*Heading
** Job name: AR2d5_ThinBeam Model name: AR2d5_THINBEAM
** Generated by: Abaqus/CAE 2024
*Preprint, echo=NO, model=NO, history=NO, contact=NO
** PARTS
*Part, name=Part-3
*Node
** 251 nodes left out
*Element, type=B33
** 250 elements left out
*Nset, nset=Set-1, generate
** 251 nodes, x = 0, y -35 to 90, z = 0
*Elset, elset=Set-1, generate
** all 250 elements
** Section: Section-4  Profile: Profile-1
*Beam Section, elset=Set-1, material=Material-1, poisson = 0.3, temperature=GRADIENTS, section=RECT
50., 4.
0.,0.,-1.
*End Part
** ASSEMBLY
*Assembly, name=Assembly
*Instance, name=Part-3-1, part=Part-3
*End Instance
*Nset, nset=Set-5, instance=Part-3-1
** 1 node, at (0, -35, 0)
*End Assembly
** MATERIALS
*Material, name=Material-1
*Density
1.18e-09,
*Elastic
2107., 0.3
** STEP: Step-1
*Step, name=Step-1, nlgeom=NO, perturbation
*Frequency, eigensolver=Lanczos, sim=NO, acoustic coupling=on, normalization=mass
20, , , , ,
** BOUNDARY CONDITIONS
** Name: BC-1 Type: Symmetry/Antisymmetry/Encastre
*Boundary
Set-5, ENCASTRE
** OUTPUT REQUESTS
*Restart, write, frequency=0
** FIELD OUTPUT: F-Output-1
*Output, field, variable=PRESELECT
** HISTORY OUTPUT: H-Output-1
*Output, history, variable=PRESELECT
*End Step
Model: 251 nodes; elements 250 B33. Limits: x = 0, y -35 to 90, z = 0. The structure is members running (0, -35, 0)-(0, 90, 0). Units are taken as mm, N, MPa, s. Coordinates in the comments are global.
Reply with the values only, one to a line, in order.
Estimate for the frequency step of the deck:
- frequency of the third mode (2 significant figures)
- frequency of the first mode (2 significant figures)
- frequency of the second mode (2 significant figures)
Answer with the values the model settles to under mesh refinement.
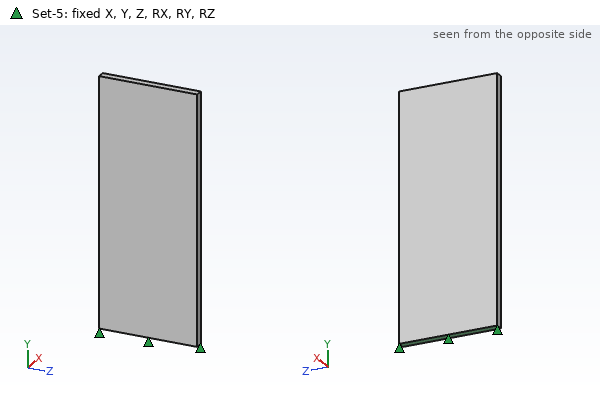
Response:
350 Hz
57 Hz
260 Hz
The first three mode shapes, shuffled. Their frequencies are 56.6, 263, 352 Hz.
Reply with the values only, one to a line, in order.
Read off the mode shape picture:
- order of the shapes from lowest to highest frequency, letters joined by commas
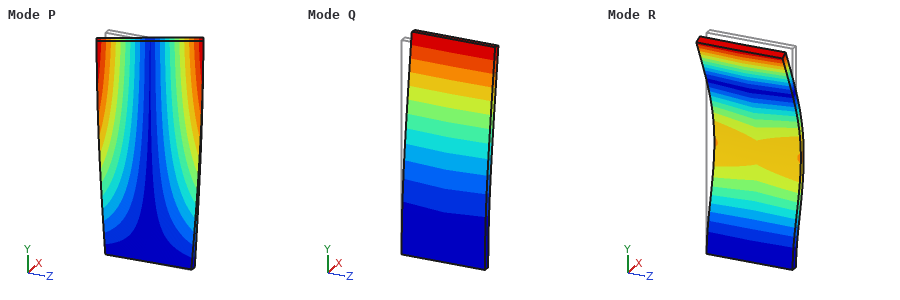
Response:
Q, P, R
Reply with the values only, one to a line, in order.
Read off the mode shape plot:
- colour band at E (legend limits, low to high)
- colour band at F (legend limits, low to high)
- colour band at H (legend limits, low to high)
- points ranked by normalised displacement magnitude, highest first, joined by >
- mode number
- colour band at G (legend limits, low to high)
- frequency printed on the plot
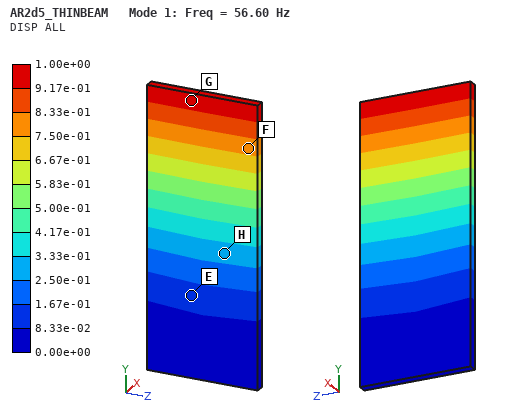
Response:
8.33e-02 to 1.67e-01
7.50e-01 to 8.33e-01
2.50e-01 to 3.33e-01
G > F > H > E
1
9.17e-01 to 1.00e+00
56.60 Hz
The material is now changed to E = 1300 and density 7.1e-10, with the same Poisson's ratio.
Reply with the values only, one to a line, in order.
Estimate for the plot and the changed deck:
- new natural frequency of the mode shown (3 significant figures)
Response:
57.3 Hz
